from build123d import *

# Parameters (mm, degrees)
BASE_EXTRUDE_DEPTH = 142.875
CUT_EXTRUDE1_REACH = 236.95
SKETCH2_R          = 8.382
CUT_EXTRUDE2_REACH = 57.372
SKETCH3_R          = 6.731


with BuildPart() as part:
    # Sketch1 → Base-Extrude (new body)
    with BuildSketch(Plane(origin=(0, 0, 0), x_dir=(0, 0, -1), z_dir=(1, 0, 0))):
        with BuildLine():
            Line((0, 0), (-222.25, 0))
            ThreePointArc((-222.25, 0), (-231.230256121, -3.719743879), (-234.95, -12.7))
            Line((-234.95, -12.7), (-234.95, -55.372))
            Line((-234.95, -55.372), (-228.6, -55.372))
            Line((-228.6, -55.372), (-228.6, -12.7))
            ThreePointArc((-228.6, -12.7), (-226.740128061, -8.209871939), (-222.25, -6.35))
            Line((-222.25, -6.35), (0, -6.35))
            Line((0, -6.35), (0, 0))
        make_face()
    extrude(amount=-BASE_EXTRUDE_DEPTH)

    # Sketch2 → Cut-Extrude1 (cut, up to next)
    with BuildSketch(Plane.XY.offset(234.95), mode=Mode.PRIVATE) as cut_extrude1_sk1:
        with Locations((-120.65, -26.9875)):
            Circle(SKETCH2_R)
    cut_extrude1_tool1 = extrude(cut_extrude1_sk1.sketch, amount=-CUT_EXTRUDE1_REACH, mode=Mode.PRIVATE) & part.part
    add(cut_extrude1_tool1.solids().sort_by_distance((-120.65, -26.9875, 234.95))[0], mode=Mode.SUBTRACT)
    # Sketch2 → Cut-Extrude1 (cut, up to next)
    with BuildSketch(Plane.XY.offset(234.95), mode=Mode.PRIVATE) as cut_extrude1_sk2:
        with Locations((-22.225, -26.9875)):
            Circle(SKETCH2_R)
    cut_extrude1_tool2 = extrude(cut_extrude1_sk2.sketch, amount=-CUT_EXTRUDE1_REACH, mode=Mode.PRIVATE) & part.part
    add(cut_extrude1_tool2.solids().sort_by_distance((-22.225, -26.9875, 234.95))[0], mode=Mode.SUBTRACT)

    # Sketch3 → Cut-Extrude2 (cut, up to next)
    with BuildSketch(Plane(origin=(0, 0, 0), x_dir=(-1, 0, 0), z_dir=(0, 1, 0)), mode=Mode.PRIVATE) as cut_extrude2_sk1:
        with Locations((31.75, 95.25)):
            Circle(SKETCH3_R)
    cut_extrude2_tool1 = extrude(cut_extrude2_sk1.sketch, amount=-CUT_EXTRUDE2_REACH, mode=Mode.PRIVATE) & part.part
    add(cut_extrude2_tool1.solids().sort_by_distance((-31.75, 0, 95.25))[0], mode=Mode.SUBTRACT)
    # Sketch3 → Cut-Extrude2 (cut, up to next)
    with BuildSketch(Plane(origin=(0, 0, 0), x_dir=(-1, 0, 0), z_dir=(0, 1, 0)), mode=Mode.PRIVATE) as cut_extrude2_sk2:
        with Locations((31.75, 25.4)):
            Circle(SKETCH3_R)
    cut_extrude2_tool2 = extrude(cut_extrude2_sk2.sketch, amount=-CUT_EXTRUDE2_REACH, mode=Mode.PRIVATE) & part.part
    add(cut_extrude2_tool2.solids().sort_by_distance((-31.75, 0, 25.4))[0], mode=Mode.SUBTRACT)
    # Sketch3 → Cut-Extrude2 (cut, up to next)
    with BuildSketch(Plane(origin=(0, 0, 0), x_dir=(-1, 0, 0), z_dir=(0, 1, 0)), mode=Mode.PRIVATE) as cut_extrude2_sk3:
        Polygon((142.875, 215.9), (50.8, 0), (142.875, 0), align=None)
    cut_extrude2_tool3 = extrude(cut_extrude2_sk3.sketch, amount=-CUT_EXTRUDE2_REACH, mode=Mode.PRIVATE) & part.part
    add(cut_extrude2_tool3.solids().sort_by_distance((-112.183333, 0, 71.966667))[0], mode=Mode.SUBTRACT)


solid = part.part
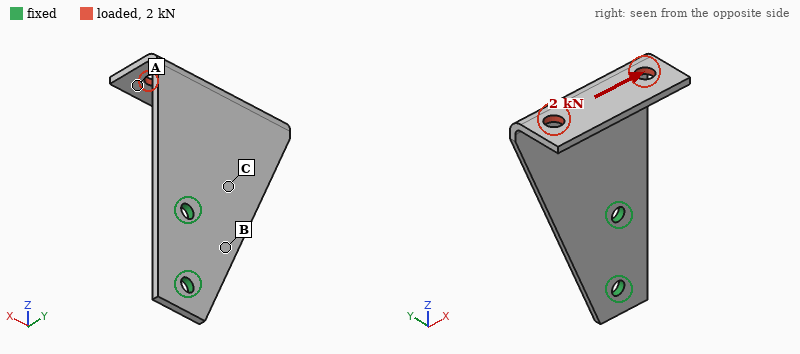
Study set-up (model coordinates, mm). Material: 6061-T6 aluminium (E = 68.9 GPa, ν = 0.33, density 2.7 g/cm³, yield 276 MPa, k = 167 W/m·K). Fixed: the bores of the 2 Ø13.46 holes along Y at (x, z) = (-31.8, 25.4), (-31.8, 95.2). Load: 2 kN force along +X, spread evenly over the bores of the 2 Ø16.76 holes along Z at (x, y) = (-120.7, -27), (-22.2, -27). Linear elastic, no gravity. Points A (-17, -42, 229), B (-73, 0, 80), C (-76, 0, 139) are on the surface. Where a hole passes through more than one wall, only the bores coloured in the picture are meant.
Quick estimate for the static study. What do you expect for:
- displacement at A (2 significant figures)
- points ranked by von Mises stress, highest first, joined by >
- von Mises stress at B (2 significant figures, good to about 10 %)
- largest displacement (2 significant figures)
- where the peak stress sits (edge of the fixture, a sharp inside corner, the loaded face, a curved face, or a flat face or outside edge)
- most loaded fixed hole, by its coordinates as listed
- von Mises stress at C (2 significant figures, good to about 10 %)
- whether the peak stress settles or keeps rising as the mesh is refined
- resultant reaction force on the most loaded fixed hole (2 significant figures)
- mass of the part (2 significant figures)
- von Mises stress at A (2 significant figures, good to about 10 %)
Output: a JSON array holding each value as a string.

["1.3 mm", "B > C > A", "64 MPa", "3.0 mm", "edge of the fixture", "(-31.8, 95.2)", "40 MPa", "keeps rising", "5.2 kN", "500 g", "13 MPa"]
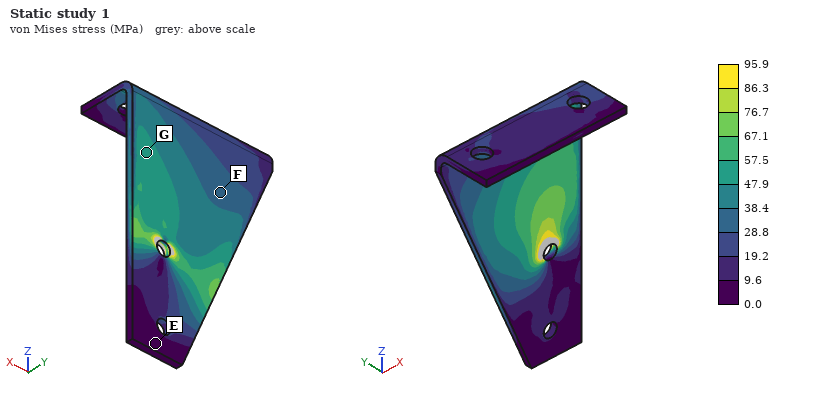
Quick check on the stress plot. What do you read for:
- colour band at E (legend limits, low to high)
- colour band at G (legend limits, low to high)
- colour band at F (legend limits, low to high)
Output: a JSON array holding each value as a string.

["0.0 to 9.6 MPa", "47.9 to 57.5 MPa", "28.8 to 38.4 MPa"]
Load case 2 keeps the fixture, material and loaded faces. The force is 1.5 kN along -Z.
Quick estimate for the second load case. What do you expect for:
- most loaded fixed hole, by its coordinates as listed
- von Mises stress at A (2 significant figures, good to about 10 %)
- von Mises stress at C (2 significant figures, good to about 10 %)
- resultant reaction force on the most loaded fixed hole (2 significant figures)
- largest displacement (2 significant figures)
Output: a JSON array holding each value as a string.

["(-31.8, 95.2)", "11 MPa", "43 MPa", "1.2 kN", "2.9 mm"]
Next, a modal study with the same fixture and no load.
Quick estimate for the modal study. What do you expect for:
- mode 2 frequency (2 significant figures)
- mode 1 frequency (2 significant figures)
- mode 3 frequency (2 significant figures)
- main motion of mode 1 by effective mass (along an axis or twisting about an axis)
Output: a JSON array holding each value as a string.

["320 Hz", "140 Hz", "770 Hz", "along Y"]
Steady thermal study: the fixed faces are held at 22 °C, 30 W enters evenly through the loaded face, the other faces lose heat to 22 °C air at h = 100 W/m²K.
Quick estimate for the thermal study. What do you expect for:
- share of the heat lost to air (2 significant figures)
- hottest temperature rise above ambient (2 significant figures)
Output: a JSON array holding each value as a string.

["90 %", "13 K"]
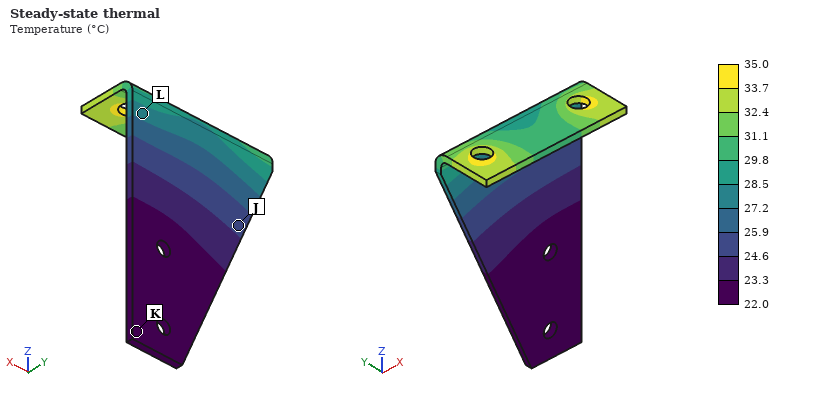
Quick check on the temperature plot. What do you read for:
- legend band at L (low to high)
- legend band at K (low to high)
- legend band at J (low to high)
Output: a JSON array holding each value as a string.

["27.2 to 28.5 °C", "22.0 to 23.3 °C", "24.6 to 25.9 °C"]
